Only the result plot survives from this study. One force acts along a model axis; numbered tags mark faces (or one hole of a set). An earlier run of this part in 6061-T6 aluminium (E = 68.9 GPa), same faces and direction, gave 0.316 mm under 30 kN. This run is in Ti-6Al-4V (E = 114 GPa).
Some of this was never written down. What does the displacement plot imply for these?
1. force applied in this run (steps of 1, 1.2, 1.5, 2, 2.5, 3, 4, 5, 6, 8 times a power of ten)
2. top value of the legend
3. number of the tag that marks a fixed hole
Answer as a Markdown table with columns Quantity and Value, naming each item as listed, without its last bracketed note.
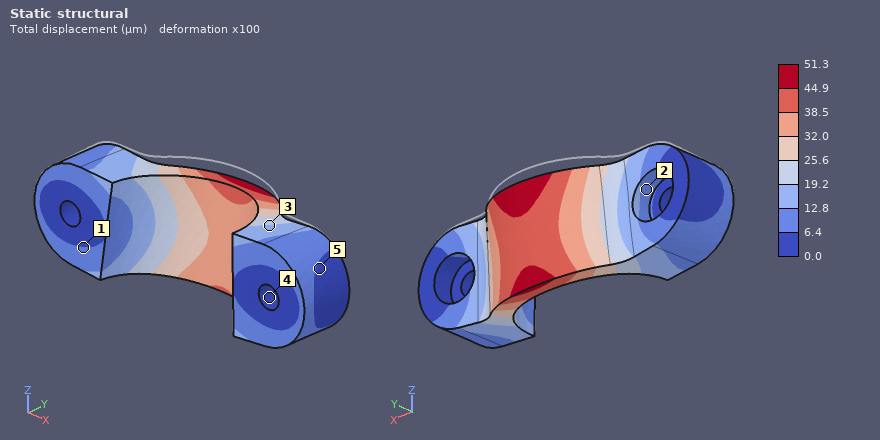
| Quantity | Value |
|---|---|
| force applied in this run | 8 kN |
| top value of the legend | 51.3 µm |
| number of the tag that marks a fixed hole | 4 |
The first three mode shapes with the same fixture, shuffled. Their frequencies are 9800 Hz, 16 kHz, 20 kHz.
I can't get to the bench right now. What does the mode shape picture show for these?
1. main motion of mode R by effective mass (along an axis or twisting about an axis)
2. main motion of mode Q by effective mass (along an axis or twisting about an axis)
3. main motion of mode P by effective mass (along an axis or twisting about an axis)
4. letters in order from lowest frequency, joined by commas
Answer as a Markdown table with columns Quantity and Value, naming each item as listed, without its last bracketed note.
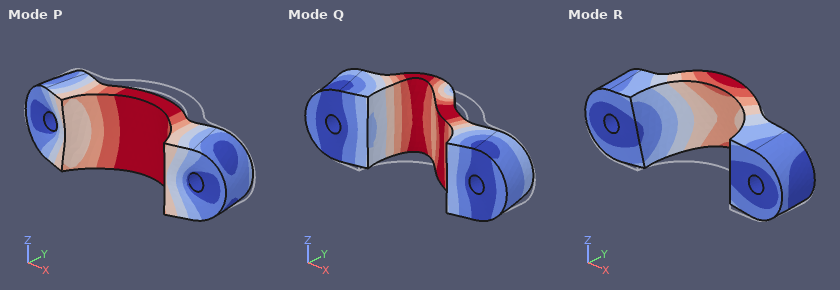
| Quantity | Value |
|---|---|
| main motion of mode R by effective mass | along Z |
| main motion of mode Q by effective mass | along X |
| main motion of mode P by effective mass | along Y |
| letters in order from lowest frequency, joined by commas | R, Q, P |
